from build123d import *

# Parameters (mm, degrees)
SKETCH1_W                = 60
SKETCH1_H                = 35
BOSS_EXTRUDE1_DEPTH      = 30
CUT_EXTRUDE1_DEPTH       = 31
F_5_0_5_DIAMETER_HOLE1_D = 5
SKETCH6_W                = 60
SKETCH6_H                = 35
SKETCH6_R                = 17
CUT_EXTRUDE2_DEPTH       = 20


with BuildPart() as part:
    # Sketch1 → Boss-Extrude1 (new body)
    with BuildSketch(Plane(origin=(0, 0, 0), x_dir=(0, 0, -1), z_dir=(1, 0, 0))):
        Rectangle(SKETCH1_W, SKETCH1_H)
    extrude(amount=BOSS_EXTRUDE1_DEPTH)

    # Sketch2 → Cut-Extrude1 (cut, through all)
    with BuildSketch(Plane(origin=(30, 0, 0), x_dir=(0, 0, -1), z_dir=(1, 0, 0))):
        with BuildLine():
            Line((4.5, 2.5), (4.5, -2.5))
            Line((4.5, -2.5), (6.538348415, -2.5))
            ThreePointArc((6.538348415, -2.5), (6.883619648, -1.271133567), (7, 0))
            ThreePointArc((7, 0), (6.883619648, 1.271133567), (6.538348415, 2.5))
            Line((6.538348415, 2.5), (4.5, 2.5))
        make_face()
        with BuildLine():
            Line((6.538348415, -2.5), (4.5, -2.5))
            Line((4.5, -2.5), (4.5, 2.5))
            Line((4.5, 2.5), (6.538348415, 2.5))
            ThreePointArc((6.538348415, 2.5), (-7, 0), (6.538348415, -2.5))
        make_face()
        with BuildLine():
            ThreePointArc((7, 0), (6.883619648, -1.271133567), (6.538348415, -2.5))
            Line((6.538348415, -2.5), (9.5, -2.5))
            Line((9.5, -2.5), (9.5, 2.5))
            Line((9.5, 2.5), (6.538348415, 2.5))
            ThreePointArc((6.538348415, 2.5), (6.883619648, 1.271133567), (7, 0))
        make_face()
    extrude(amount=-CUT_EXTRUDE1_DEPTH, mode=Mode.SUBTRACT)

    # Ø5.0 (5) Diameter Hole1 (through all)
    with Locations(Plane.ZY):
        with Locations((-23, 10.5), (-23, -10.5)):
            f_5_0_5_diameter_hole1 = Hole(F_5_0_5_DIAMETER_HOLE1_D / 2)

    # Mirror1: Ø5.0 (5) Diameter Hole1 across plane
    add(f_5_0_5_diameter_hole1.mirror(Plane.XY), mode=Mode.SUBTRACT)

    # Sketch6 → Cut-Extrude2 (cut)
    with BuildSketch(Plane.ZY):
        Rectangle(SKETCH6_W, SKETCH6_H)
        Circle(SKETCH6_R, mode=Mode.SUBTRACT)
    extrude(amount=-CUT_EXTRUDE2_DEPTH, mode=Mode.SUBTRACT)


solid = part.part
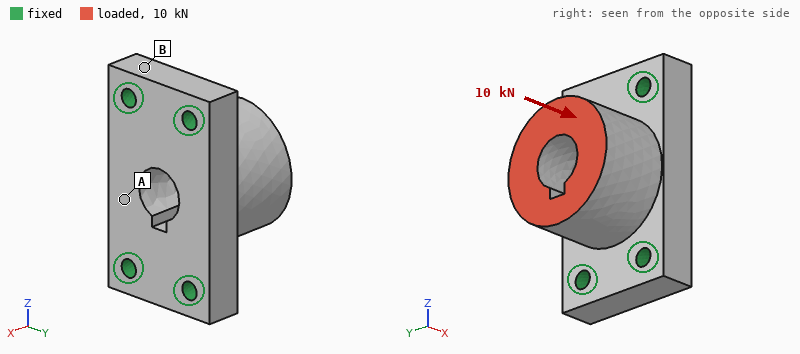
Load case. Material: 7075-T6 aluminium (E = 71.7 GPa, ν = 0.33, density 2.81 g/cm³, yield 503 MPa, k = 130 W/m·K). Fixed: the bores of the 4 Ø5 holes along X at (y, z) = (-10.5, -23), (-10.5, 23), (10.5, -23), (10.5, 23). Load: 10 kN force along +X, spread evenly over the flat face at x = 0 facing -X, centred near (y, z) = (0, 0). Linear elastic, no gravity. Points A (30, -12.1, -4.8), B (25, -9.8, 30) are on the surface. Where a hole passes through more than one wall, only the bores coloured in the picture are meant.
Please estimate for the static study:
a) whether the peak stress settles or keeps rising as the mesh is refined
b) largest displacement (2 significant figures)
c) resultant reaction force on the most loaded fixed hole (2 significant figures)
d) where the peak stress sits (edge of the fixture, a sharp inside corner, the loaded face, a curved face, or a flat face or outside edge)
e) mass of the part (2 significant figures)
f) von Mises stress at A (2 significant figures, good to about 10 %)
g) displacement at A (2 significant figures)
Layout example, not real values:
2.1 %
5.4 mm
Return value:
keeps rising
17 µm
2.7 kN
edge of the fixture
94 g
22 MPa
13 µm
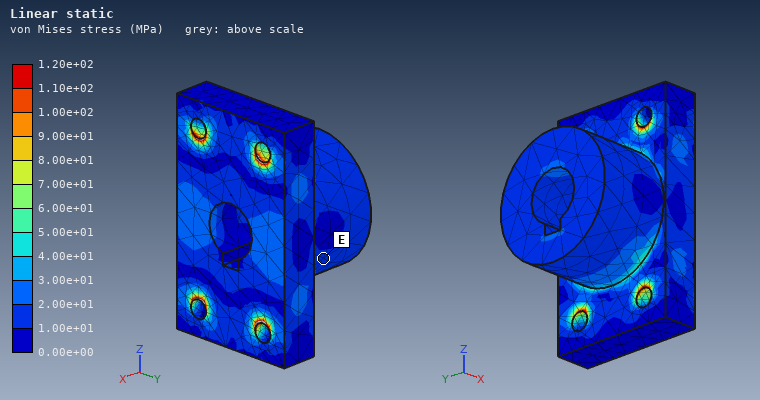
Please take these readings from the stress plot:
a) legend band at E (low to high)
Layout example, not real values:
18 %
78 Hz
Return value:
1.00e+01 to 2.00e+01 MPa
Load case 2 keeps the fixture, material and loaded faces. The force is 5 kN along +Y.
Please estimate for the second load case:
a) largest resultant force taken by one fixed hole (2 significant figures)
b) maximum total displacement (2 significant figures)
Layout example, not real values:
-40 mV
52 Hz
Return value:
3.1 kN
54 µm
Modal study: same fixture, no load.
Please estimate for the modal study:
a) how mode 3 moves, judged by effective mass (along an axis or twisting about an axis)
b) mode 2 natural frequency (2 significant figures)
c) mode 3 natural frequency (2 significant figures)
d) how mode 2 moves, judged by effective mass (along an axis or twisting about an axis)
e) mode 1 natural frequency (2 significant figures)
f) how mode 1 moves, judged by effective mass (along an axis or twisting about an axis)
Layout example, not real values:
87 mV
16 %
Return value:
along Z
17 kHz
18 kHz
along X
11 kHz
along Y
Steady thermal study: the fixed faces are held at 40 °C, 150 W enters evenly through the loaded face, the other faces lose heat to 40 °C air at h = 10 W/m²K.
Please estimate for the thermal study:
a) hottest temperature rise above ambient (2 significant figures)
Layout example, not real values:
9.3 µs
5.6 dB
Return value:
55 K
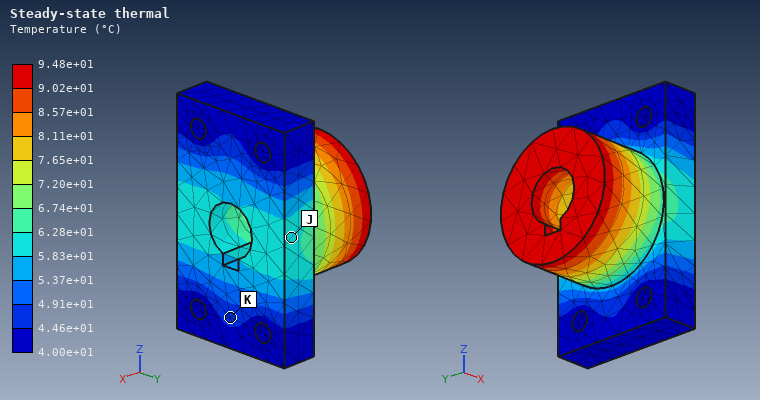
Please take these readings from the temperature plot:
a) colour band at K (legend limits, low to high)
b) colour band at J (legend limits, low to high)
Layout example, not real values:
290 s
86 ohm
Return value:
4.46e+01 to 4.91e+01 °C
5.83e+01 to 6.28e+01 °C
